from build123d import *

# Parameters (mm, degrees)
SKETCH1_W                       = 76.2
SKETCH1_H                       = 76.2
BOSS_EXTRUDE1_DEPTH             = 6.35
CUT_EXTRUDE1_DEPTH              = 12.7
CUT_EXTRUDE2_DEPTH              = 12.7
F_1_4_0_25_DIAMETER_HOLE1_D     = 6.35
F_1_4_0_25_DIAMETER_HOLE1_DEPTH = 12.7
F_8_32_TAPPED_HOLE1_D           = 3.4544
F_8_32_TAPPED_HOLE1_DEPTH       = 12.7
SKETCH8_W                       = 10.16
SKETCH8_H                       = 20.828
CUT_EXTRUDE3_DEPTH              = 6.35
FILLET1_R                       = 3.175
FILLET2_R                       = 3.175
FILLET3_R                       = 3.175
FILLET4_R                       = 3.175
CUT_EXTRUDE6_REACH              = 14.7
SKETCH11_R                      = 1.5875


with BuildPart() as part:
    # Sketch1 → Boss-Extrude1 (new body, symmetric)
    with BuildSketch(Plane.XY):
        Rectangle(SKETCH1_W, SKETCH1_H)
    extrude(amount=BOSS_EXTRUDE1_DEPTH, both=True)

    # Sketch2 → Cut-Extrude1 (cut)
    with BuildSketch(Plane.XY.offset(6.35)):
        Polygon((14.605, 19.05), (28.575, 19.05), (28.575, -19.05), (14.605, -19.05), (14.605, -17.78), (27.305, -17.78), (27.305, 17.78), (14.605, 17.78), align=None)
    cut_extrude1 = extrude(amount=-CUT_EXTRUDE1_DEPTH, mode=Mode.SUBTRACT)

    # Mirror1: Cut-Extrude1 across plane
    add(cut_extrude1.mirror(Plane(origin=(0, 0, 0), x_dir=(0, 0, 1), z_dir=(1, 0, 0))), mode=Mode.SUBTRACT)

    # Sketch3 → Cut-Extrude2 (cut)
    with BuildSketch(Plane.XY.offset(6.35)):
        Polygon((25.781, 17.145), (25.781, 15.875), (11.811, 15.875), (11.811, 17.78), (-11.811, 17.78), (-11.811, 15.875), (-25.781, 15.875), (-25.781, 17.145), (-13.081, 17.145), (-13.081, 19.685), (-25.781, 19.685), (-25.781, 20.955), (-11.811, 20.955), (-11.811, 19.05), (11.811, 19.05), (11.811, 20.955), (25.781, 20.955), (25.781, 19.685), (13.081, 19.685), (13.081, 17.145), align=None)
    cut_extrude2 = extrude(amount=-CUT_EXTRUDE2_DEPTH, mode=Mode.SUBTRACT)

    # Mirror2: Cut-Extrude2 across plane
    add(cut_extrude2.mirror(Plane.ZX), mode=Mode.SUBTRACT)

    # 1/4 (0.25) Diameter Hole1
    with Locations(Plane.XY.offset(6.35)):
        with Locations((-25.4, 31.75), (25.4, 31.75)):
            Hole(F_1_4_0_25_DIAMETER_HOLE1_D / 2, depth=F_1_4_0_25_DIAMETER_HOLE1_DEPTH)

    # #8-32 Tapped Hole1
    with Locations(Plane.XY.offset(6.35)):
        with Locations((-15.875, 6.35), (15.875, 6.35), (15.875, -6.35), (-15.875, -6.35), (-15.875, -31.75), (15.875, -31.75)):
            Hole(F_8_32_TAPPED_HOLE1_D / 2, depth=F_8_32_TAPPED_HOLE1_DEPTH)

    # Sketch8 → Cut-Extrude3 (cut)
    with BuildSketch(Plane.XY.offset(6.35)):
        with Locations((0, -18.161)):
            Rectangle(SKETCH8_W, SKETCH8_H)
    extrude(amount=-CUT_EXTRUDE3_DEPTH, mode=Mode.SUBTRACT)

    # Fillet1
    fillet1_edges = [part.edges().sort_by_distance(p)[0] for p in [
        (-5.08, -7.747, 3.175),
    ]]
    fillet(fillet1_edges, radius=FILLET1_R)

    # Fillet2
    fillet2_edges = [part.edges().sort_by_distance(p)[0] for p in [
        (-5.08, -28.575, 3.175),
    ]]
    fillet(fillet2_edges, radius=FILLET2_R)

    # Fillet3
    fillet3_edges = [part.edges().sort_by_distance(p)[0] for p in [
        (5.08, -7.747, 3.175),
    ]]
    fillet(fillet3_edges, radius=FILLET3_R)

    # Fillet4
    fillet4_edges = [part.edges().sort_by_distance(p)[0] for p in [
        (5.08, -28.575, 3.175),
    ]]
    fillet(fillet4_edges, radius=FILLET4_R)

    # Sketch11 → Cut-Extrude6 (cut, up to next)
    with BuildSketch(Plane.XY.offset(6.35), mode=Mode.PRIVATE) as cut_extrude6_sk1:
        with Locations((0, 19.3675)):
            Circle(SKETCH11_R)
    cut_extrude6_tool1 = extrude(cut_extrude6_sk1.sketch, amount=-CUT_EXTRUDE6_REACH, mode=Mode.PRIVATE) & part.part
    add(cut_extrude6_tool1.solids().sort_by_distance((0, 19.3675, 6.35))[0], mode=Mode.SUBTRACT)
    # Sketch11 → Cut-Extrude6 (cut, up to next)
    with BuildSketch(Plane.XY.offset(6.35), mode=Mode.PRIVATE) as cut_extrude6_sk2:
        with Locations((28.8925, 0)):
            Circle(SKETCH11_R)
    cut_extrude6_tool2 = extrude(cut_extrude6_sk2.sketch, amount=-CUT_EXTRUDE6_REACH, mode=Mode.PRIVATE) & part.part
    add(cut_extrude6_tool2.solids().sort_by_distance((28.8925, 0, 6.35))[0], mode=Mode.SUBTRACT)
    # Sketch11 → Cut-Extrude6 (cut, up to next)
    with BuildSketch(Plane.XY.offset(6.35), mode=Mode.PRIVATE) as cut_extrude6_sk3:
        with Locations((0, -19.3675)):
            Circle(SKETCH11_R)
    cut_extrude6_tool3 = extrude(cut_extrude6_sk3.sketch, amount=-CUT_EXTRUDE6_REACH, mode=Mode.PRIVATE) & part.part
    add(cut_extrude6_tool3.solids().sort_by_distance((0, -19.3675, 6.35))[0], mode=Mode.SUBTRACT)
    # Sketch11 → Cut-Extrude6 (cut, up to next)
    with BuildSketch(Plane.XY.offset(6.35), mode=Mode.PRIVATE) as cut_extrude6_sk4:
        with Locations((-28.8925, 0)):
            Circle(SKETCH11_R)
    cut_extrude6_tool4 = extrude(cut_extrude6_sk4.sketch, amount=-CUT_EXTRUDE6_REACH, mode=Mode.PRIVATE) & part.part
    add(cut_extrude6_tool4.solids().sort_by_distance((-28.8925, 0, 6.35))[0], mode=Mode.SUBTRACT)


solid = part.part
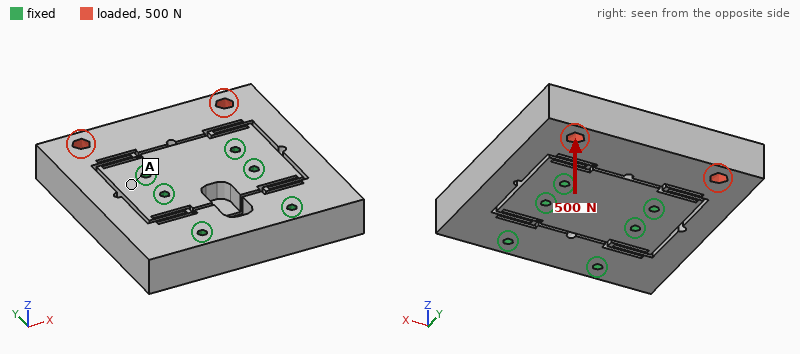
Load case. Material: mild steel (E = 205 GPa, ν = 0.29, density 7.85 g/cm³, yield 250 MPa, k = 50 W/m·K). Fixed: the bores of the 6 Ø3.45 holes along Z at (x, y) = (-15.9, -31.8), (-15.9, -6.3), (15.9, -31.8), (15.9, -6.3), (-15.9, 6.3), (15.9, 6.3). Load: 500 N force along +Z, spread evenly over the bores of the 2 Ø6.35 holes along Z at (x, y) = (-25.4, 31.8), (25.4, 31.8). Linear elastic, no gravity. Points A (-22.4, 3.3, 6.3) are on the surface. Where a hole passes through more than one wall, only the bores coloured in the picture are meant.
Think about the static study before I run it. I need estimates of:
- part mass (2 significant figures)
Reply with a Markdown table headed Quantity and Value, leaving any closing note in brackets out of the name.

| Quantity | Value |
|---|---|
| part mass | 520 g |
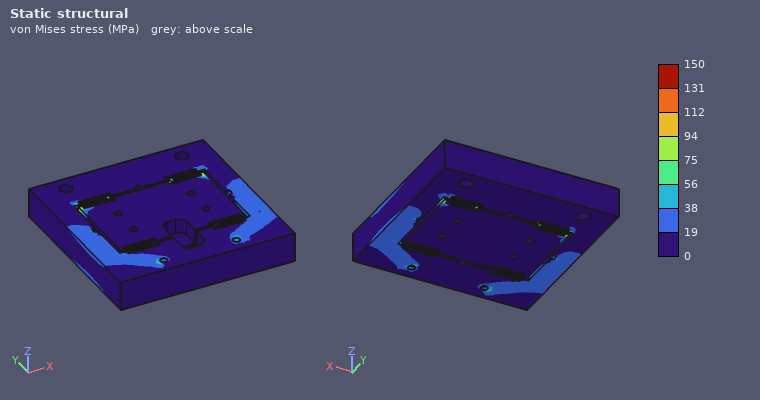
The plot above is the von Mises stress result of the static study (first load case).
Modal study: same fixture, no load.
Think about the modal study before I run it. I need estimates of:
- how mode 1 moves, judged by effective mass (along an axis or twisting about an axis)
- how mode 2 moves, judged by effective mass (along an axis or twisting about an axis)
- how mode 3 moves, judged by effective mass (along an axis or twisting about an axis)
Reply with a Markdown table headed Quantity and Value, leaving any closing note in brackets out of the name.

| Quantity | Value |
|---|---|
| how mode 1 moves, judged by effective mass | along Z |
| how mode 2 moves, judged by effective mass | along X |
| how mode 3 moves, judged by effective mass | twisting about Y |
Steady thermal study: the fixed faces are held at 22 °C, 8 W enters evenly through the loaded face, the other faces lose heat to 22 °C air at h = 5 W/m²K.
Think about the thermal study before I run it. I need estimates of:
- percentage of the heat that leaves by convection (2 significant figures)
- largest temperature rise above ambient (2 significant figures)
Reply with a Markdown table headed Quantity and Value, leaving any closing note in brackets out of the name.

| Quantity | Value |
|---|---|
| percentage of the heat that leaves by convection | 16 % |
| largest temperature rise above ambient | 33 K |
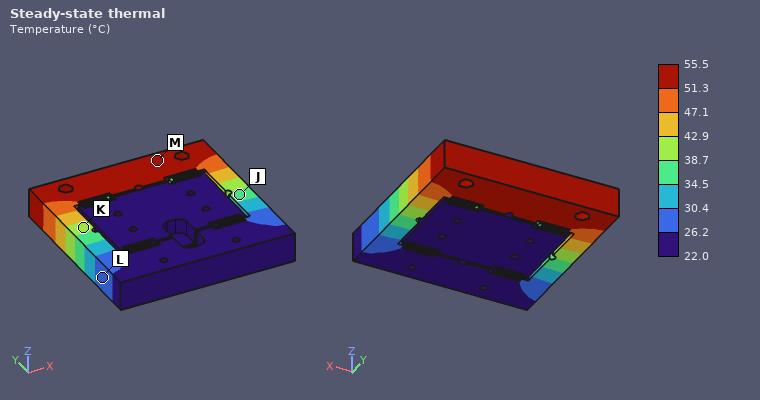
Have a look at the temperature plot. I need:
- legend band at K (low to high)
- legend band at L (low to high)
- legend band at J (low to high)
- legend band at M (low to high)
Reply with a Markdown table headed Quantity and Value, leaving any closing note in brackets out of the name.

| Quantity | Value |
|---|---|
| legend band at K | 38.7 to 42.9 °C |
| legend band at L | 26.2 to 30.4 °C |
| legend band at J | 34.5 to 38.7 °C |
| legend band at M | 51.3 to 55.5 °C |
